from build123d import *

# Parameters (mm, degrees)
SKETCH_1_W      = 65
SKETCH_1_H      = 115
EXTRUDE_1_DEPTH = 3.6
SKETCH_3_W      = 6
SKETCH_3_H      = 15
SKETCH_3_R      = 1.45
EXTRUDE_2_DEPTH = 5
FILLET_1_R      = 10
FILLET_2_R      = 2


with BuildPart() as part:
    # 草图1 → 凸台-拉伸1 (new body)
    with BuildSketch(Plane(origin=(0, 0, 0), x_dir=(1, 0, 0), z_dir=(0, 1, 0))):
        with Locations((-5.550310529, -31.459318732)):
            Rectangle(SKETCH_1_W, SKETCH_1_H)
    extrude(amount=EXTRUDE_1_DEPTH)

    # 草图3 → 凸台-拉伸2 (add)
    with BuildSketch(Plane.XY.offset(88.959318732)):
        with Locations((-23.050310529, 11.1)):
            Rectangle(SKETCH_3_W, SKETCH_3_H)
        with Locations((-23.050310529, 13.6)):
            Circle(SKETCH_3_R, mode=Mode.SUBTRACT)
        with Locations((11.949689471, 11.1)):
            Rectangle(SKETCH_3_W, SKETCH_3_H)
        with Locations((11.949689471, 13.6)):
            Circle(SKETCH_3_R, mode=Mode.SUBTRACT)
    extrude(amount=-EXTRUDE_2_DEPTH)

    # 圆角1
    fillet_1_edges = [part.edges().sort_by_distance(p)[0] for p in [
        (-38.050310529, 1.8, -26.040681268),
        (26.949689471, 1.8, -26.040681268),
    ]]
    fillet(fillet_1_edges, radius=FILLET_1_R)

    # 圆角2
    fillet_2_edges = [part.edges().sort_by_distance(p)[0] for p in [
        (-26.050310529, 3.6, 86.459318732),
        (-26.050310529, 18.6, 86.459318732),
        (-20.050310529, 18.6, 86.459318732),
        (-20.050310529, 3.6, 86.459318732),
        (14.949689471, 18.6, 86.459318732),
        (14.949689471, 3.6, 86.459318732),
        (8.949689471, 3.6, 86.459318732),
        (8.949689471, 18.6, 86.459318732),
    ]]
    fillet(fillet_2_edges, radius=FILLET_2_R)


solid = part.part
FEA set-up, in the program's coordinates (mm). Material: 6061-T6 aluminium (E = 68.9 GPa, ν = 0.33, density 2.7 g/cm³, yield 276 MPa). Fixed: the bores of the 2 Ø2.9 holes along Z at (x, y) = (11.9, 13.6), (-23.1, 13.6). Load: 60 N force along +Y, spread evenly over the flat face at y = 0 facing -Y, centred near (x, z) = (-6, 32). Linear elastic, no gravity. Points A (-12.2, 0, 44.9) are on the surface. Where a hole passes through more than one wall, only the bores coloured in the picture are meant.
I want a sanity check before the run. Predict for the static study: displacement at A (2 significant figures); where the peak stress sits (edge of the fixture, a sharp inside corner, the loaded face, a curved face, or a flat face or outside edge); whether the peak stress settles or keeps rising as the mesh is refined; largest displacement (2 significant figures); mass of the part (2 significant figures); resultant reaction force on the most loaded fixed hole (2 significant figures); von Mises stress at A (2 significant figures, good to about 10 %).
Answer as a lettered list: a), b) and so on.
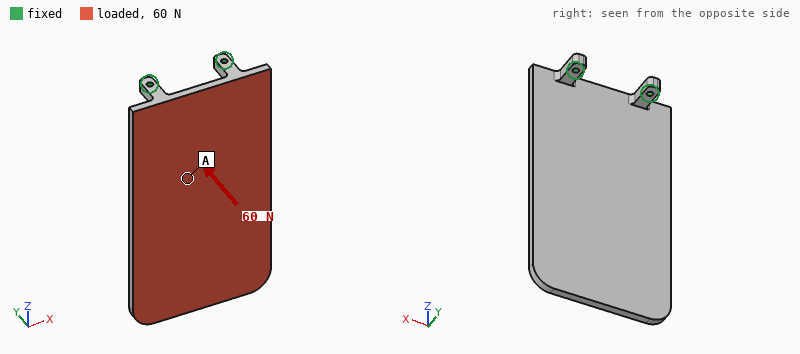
a) 0.31 mm
b) edge of the fixture
c) keeps rising
d) 1.1 mm
e) 74 g
f) 35 N
g) 8.8 MPa
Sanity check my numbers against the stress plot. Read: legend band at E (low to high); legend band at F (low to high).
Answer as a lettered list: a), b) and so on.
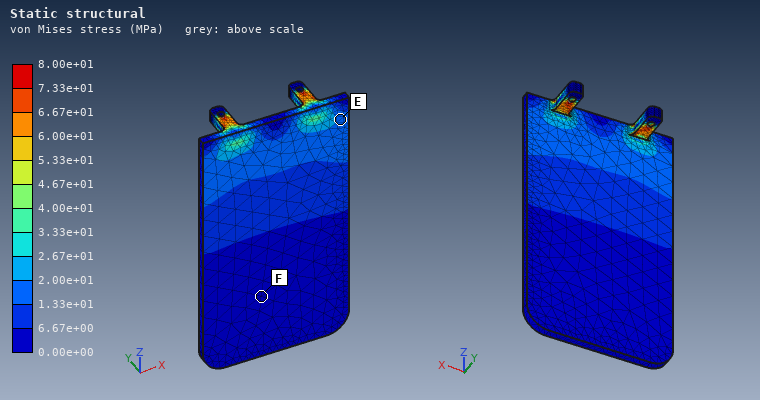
a) 1.33e+01 to 2.00e+01 MPa
b) 0.00e+00 to 6.67e+00 MPa
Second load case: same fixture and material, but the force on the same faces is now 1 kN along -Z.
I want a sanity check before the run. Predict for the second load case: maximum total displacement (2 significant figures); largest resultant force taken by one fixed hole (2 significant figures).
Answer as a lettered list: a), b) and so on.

a) 1.5 mm
b) 500 N
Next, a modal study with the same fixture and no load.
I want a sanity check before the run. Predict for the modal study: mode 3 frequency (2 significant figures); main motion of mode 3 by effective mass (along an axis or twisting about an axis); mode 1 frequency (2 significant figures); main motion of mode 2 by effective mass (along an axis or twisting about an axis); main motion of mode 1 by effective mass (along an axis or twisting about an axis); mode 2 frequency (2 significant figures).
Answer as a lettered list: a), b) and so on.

a) 930 Hz
b) along X
c) 170 Hz
d) along X
e) along Y
f) 730 Hz
